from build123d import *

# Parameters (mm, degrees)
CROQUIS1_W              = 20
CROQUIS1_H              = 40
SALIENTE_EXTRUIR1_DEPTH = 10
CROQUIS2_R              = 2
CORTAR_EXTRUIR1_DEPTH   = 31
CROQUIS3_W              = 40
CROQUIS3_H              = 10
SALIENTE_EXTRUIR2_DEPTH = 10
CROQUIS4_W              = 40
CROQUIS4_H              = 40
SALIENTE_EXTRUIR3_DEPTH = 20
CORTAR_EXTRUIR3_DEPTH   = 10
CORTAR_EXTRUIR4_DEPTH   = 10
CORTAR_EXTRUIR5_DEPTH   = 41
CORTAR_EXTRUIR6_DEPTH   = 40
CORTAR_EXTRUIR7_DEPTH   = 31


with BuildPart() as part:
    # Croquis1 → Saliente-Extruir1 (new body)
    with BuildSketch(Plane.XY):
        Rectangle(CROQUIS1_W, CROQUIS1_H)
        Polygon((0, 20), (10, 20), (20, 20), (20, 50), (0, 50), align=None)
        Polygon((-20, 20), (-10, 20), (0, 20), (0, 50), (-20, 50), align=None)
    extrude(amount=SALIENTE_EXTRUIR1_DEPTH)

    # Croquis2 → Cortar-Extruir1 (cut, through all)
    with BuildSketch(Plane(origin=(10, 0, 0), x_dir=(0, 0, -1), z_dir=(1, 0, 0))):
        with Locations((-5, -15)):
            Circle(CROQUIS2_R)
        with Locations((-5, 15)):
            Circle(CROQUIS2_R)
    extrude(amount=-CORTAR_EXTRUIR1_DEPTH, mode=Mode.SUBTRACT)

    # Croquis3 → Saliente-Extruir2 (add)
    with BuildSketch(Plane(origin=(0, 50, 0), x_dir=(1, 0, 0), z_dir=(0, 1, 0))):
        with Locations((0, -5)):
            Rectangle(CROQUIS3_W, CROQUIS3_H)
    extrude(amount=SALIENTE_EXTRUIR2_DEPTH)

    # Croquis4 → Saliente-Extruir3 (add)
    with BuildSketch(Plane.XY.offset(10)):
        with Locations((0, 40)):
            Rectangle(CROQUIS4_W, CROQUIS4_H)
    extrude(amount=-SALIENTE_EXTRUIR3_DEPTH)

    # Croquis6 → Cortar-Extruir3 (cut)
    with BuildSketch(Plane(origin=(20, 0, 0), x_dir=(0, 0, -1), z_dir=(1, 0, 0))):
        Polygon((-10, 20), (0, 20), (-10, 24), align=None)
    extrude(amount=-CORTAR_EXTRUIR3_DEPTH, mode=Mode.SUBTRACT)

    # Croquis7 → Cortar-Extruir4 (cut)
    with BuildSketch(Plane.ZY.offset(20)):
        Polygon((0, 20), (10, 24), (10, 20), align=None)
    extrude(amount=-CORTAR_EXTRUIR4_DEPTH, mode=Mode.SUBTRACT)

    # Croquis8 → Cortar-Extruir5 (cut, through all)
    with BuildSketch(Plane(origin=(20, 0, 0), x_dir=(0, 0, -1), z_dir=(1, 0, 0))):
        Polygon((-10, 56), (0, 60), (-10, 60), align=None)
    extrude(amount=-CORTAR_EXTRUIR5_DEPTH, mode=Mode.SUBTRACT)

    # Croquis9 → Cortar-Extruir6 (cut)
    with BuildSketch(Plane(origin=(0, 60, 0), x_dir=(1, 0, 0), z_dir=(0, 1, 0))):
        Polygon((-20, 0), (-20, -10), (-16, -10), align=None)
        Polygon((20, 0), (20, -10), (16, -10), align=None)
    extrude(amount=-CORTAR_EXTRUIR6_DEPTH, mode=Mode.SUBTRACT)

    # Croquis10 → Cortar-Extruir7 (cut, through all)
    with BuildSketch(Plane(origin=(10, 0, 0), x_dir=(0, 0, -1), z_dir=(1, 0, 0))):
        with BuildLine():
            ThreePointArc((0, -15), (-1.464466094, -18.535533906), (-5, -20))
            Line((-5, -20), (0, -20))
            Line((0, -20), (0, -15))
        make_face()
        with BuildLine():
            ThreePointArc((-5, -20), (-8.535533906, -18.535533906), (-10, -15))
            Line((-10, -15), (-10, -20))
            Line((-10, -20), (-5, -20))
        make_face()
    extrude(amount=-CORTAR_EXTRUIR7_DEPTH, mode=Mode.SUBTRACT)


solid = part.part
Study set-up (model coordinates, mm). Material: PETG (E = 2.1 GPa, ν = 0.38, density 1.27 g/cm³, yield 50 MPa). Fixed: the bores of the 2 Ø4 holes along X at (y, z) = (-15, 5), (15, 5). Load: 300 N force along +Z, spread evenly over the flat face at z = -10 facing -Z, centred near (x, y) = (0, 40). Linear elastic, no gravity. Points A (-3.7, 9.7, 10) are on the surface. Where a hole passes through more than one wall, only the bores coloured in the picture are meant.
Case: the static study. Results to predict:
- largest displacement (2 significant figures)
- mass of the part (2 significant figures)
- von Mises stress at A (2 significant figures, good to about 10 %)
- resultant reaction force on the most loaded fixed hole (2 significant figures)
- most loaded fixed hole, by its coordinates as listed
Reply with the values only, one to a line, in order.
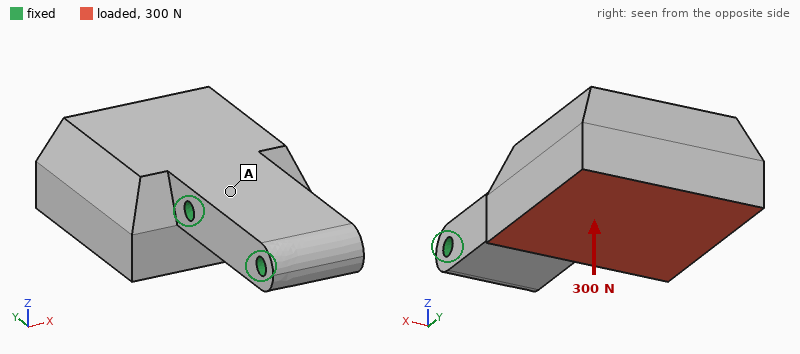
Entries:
0.93 mm
47 g
4.0 MPa
380 N
(15, 5)
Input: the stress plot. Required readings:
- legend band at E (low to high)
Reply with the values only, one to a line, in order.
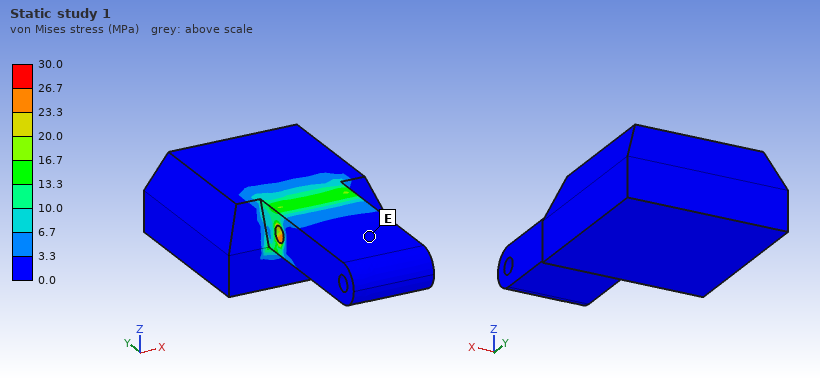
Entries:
0.0 to 3.3 MPa
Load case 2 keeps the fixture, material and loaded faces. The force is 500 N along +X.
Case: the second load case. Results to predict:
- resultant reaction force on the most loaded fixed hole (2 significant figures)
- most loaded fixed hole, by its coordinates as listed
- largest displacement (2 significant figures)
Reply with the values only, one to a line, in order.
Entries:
520 N
(15, 5)
0.54 mm
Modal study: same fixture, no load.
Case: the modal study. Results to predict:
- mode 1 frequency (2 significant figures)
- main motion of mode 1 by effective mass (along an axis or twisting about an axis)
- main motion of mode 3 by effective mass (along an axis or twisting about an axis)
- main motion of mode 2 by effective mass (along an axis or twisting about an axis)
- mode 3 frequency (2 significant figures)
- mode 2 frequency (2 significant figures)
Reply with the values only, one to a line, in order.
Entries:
570 Hz
along Z
twisting about Y
along X
1500 Hz
1100 Hz
